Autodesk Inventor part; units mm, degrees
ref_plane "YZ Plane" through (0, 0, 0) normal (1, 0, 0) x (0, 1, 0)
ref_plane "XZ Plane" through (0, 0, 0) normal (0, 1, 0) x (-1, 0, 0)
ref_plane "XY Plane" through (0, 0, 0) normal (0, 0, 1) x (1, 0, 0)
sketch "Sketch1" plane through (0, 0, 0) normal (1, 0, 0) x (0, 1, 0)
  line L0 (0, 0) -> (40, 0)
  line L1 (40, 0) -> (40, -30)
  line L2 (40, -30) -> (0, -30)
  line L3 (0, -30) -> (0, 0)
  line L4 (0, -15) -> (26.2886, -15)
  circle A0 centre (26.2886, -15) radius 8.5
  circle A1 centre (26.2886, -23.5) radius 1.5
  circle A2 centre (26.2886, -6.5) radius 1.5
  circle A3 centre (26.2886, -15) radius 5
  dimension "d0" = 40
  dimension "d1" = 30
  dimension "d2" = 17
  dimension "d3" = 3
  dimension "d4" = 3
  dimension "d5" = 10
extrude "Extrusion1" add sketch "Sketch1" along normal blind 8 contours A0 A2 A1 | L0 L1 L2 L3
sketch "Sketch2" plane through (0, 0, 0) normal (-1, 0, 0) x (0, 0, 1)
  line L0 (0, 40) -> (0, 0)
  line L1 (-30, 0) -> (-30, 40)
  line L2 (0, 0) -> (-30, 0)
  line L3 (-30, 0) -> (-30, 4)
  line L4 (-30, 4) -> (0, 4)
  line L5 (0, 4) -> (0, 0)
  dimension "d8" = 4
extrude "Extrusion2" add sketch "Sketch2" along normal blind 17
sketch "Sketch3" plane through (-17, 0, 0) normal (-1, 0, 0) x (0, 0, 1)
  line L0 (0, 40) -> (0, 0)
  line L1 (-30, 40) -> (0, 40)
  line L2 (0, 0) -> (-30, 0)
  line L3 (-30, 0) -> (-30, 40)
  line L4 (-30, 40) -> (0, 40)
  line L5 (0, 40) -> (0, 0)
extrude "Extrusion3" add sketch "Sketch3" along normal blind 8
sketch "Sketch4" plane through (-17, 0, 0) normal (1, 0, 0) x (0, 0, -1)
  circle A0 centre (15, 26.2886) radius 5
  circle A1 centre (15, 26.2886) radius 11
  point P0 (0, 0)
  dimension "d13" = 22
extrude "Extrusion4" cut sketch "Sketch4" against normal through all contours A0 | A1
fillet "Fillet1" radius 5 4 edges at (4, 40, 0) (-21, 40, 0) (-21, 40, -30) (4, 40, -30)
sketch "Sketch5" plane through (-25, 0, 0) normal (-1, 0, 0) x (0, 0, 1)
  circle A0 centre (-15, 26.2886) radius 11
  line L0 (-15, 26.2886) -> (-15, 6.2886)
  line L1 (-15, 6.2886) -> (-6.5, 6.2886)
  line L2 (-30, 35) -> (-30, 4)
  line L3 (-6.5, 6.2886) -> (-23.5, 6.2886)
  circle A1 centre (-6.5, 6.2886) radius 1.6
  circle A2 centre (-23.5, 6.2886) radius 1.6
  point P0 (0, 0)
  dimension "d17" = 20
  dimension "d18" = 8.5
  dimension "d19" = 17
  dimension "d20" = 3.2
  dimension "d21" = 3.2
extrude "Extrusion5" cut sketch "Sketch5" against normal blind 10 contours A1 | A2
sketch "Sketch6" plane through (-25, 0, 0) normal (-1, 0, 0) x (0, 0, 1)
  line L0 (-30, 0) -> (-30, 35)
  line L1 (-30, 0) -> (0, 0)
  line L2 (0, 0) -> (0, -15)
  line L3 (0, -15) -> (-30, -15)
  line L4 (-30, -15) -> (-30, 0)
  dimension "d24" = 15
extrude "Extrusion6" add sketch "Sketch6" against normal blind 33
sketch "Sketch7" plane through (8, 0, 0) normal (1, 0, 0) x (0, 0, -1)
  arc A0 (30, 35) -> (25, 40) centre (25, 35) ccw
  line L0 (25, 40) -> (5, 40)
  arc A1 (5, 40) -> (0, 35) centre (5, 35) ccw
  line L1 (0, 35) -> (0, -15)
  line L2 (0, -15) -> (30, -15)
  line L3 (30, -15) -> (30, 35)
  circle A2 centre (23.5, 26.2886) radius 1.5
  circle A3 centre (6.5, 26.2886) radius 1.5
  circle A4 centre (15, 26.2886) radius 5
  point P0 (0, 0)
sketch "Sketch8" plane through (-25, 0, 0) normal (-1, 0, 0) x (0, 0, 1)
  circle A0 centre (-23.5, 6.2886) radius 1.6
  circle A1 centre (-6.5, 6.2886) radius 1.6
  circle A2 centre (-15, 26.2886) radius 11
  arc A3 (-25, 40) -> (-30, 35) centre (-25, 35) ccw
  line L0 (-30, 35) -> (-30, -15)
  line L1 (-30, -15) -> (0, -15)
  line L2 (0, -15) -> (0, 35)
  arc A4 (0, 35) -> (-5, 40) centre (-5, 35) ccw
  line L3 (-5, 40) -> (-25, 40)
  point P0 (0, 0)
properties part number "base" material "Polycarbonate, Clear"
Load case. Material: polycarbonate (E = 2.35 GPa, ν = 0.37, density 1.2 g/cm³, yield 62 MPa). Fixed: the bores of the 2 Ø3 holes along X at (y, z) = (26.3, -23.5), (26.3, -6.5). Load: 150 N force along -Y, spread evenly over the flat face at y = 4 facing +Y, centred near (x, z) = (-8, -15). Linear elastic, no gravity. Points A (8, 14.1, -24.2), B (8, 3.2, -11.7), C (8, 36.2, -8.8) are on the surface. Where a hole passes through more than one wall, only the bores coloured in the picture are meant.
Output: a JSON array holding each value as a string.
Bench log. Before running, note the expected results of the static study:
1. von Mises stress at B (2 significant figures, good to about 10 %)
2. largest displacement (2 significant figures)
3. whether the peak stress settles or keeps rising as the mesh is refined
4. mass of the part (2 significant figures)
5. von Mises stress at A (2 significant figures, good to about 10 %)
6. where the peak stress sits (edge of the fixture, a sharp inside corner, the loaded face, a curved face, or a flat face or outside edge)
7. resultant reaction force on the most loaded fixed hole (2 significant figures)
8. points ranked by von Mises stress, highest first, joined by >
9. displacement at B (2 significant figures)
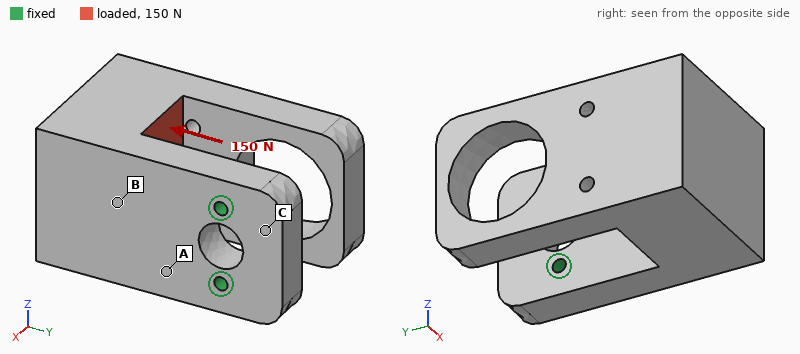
["3.8 MPa", "0.74 mm", "keeps rising", "38 g", "5.3 MPa", "edge of the fixture", "76 N", "A > B > C", "0.21 mm"]
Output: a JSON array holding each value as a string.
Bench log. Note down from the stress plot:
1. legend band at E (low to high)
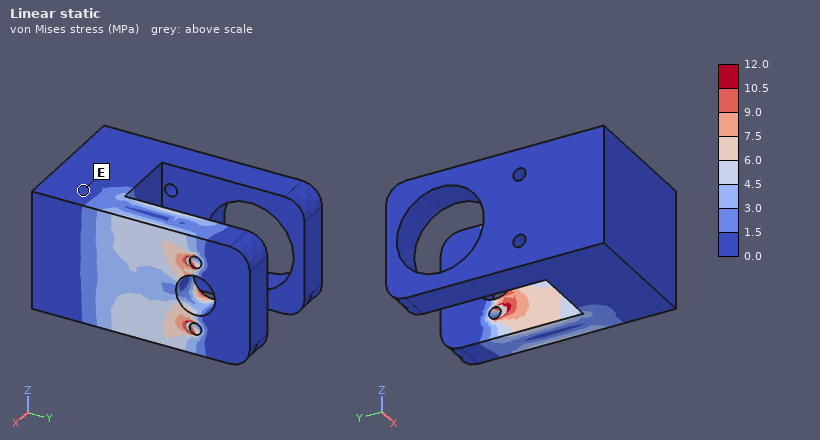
["0.0 to 1.5 MPa"]
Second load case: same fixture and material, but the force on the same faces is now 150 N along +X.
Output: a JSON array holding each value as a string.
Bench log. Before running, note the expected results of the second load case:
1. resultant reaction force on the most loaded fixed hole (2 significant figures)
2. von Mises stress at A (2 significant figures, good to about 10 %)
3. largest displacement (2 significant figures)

["75 N", "4.9 MPa", "0.70 mm"]
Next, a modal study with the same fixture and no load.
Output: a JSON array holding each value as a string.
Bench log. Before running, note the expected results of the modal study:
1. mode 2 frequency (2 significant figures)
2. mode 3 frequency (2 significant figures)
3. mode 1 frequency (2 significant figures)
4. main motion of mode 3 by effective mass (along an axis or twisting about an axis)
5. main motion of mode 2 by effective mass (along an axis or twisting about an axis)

["630 Hz", "980 Hz", "350 Hz", "along X", "along Z"]
